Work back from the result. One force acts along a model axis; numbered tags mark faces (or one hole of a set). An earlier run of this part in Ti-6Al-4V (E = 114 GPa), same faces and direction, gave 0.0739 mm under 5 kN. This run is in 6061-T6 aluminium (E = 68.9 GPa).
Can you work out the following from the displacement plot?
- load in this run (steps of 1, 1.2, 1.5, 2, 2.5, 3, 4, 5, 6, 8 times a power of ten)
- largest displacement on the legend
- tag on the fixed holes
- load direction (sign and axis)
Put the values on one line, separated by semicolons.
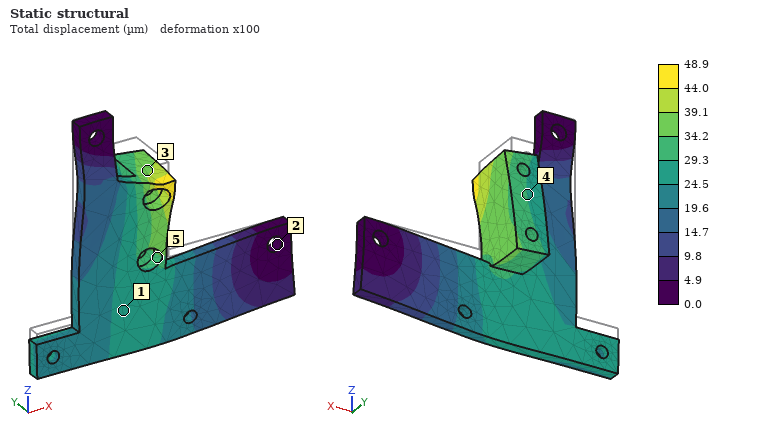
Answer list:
2 kN; 48.9 µm; 2; -Z
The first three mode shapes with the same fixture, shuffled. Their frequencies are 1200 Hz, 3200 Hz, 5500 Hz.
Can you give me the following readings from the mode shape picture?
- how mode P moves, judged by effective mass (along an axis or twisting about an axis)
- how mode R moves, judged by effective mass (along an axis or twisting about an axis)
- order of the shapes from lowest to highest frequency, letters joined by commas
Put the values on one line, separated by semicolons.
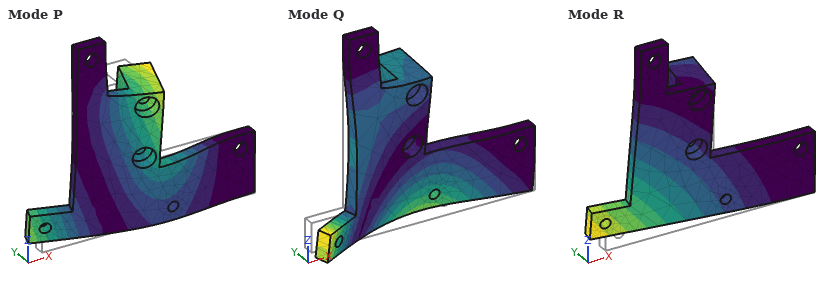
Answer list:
along Y; along Y; R, P, Q
